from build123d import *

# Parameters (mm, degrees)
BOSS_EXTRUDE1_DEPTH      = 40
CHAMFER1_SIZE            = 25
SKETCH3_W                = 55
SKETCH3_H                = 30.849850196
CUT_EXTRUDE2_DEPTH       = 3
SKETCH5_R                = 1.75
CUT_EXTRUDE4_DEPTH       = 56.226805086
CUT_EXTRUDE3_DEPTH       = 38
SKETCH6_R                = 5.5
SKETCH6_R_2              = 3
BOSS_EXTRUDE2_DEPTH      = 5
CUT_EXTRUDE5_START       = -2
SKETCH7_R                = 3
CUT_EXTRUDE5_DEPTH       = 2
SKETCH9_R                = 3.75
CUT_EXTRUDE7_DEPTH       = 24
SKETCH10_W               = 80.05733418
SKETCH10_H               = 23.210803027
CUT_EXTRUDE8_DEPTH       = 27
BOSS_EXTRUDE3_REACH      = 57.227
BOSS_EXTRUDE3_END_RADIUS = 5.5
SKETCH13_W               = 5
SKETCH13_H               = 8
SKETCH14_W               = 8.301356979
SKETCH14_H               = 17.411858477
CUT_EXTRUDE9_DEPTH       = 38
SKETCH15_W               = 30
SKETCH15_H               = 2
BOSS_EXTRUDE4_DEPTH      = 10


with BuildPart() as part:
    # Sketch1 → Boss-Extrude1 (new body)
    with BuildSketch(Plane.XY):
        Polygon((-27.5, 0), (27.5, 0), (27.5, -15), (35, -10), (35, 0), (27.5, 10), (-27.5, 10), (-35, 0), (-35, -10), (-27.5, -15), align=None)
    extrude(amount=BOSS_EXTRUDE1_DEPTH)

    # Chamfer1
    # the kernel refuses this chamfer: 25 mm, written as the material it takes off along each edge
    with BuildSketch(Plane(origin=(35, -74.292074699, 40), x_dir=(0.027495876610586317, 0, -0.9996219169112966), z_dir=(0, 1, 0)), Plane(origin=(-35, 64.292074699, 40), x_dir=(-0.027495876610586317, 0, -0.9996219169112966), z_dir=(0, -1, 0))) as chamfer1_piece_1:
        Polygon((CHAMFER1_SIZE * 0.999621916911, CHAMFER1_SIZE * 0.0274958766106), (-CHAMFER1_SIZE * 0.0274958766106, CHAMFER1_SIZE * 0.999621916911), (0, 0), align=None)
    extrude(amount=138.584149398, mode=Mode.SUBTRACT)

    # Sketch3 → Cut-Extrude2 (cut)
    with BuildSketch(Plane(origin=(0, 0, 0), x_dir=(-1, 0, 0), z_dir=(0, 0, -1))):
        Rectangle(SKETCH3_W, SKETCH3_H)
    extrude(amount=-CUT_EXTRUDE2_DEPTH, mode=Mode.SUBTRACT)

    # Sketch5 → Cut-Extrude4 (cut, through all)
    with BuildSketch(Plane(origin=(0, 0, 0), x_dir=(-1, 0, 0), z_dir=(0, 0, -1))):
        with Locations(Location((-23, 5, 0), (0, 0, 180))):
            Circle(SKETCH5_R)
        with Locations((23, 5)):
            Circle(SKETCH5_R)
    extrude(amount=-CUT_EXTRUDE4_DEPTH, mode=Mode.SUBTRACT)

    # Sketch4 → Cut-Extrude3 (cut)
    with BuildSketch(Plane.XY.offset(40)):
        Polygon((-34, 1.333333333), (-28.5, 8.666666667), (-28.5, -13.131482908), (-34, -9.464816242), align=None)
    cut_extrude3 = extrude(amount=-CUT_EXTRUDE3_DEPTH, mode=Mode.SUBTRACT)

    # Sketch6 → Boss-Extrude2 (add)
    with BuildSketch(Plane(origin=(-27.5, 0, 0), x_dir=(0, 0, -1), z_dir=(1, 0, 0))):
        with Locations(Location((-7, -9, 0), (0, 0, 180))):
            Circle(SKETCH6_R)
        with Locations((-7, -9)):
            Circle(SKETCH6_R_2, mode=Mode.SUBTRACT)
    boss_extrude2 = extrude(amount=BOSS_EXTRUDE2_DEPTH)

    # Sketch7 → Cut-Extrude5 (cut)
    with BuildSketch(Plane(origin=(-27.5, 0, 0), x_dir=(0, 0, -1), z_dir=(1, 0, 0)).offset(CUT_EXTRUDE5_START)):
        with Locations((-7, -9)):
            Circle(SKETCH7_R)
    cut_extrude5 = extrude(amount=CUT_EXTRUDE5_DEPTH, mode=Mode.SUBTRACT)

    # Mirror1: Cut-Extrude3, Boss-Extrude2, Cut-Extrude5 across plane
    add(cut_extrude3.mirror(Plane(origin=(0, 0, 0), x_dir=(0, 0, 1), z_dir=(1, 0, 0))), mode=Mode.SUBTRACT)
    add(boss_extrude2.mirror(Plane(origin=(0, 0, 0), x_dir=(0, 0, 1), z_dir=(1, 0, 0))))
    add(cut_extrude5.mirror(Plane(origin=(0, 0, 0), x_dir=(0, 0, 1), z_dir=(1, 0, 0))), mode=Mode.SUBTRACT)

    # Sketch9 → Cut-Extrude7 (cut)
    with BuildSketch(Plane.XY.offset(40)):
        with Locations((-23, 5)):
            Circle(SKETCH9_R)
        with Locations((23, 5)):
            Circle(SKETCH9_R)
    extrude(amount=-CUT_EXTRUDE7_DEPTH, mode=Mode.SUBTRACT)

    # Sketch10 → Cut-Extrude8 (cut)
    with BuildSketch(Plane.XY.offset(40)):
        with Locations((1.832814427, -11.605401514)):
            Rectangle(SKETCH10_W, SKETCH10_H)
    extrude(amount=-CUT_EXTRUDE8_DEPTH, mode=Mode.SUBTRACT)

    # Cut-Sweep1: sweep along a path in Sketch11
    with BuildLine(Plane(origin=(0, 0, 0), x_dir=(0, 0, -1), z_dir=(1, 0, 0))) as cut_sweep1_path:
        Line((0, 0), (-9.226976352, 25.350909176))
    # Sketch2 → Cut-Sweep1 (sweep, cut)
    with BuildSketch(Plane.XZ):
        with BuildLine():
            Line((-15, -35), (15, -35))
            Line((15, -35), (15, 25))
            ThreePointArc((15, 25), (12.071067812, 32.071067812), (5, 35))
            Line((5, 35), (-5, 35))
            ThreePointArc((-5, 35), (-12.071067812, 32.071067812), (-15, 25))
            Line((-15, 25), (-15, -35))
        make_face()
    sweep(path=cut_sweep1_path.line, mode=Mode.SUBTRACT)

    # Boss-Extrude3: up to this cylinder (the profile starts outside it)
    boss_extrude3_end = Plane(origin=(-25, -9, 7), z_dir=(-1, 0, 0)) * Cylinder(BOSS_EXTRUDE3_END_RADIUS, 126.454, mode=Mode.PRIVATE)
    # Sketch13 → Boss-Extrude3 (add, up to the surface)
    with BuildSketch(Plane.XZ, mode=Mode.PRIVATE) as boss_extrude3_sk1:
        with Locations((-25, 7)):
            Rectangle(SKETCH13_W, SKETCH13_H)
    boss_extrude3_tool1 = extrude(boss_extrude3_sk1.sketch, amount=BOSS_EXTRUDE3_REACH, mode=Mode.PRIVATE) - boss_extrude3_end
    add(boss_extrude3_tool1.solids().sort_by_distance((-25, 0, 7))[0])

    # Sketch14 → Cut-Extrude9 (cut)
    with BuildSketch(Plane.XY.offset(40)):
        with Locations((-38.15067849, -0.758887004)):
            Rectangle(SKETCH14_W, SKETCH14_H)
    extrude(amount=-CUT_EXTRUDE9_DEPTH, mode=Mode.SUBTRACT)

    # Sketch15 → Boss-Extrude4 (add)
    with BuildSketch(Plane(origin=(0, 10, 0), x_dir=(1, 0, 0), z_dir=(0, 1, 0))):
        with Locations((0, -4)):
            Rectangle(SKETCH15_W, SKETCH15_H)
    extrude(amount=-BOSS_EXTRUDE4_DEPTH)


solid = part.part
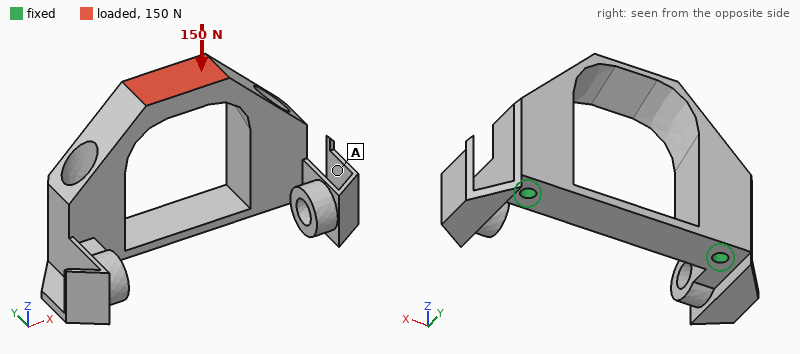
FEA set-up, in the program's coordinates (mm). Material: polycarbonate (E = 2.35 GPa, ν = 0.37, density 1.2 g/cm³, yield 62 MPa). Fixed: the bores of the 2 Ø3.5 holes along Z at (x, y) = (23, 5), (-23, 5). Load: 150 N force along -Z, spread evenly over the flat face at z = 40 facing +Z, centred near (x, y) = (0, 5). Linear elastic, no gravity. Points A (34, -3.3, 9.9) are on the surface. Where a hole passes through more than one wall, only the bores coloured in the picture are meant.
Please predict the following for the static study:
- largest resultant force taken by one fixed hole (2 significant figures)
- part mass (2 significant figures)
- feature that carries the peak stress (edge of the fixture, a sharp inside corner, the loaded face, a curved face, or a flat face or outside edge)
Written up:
98 N
11 g
the loaded face
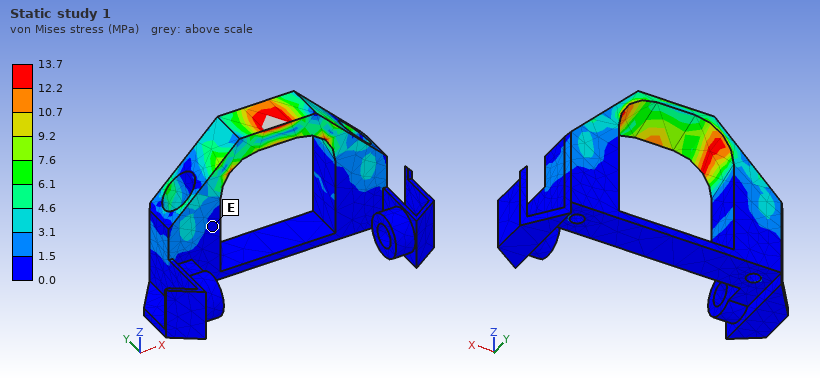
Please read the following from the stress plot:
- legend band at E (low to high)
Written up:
0.0 to 1.5 MPa
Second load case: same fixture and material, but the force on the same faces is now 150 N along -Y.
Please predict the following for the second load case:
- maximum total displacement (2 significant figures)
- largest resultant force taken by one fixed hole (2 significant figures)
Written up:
0.74 mm
76 N
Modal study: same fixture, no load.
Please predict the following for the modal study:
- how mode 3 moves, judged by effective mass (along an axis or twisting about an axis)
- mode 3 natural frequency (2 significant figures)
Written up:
along Y
2300 Hz
